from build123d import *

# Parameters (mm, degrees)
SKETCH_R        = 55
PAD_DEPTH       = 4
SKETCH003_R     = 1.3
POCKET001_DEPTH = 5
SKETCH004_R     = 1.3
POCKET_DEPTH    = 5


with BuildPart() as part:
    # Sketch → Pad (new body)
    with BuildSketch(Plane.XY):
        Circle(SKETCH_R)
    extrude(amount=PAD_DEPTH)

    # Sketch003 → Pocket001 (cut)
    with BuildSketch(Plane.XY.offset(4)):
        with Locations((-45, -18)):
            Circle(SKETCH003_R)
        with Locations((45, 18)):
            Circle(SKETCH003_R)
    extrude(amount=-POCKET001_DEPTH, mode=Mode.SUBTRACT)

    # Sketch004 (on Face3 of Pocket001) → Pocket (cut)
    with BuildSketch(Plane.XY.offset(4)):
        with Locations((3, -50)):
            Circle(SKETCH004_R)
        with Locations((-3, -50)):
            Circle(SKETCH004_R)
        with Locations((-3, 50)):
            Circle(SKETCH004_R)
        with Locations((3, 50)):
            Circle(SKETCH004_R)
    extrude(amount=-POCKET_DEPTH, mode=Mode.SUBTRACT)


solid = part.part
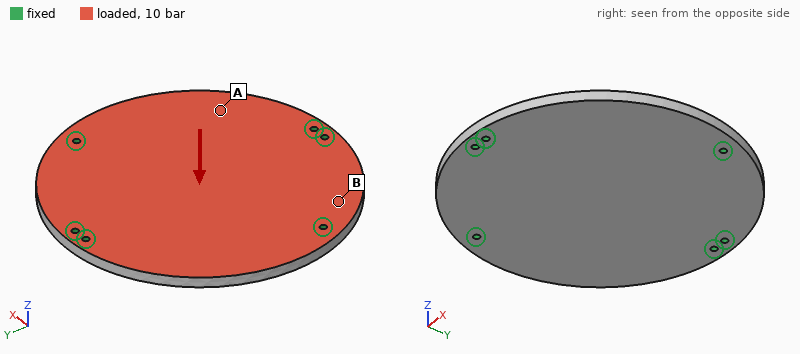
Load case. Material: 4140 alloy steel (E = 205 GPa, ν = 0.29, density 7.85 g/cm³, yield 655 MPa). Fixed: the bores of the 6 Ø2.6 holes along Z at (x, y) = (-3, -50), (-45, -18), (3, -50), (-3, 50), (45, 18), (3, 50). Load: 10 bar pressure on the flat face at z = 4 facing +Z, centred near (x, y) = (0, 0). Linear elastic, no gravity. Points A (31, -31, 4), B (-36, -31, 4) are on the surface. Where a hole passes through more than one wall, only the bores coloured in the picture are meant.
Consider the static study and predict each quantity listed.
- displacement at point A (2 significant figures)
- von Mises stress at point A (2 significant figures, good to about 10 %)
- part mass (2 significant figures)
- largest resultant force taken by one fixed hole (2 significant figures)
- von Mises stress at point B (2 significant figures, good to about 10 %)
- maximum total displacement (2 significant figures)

0.17 mm
120 MPa
300 g
2.4 kN
43 MPa
0.22 mm
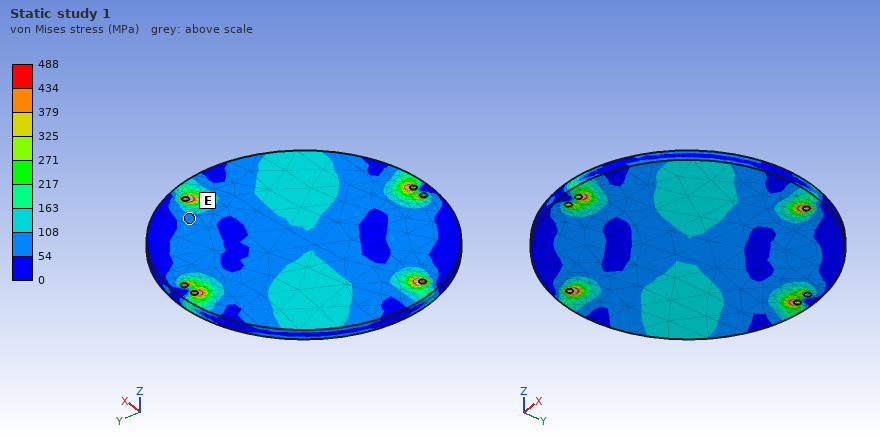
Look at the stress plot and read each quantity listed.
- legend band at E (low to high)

54 to 108 MPa
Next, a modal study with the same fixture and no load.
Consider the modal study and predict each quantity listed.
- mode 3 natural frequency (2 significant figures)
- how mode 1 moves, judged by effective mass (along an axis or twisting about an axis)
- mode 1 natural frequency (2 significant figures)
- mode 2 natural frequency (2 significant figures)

3300 Hz
along Z
2300 Hz
2500 Hz
